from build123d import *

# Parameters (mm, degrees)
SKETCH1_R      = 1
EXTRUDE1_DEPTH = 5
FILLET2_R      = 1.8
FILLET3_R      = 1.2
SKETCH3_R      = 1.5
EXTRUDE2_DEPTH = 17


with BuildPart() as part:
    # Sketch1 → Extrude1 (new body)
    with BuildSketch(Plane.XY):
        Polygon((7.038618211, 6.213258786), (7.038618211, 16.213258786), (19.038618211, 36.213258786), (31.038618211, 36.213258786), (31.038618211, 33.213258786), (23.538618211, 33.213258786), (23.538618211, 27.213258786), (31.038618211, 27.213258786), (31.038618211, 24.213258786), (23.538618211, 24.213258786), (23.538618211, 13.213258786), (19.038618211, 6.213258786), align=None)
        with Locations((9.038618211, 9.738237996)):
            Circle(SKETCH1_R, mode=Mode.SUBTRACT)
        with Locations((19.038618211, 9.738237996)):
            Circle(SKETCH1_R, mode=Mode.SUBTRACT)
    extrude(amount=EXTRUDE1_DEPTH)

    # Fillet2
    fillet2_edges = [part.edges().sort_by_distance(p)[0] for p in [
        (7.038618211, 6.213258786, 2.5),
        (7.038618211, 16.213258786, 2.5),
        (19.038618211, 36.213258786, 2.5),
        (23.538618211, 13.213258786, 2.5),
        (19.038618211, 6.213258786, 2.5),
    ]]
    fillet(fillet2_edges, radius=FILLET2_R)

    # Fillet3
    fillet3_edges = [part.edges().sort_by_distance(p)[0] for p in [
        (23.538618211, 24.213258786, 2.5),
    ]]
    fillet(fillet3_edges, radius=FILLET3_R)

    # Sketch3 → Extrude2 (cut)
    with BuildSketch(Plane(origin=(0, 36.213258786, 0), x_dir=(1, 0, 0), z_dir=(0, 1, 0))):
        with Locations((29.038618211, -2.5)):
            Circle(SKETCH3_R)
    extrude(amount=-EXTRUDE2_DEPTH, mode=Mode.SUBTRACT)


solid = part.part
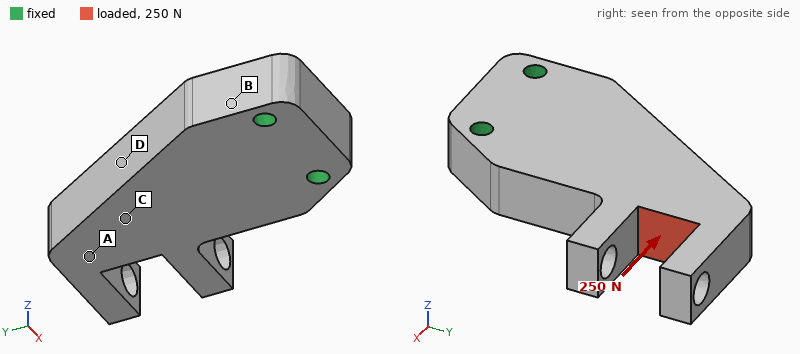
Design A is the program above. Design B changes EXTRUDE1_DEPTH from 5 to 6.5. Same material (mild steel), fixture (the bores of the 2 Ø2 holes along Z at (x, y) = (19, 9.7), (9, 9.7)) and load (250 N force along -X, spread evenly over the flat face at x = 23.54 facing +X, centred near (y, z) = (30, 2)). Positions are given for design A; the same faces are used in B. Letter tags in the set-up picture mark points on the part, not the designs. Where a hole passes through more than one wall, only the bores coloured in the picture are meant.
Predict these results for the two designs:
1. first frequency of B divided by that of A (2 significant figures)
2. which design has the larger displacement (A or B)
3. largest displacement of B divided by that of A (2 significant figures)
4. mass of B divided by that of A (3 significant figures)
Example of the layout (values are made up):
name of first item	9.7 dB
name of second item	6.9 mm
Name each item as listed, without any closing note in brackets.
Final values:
first frequency of B divided by that of A	1.2
which design has the larger displacement	A
largest displacement of B divided by that of A	0.77
mass of B divided by that of A	1.31
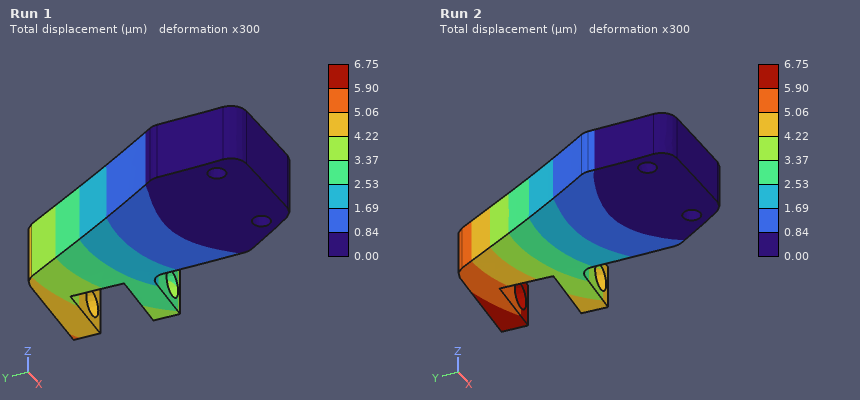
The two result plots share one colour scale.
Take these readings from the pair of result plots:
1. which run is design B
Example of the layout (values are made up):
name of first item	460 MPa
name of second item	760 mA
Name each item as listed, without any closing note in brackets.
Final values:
which run is design B	Run 1
